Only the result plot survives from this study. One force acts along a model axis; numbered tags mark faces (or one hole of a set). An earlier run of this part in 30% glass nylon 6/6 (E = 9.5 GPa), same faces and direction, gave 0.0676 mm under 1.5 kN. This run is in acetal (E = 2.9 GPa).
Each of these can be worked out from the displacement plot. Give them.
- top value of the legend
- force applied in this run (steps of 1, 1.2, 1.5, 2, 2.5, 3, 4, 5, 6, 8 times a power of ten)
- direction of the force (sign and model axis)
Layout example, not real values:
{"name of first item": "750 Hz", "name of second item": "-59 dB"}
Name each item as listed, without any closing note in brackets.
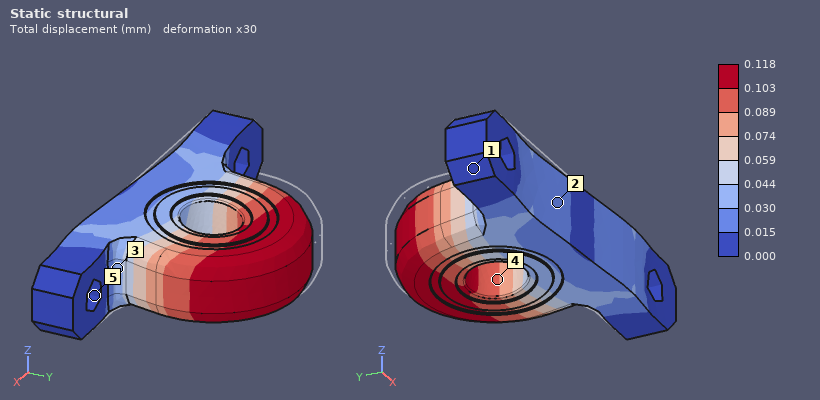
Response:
{"top value of the legend": "0.118 mm", "force applied in this run": "800 N", "direction of the force": "+X"}
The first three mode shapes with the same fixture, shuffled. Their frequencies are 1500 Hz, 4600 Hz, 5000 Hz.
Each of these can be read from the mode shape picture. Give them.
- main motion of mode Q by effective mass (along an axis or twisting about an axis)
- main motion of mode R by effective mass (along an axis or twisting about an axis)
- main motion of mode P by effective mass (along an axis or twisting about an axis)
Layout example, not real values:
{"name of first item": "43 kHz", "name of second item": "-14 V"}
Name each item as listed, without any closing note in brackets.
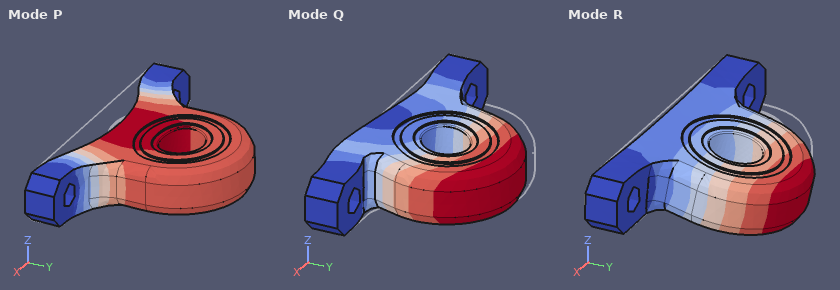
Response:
{"main motion of mode Q by effective mass": "along X", "main motion of mode R by effective mass": "along Z", "main motion of mode P by effective mass": "along Y"}
